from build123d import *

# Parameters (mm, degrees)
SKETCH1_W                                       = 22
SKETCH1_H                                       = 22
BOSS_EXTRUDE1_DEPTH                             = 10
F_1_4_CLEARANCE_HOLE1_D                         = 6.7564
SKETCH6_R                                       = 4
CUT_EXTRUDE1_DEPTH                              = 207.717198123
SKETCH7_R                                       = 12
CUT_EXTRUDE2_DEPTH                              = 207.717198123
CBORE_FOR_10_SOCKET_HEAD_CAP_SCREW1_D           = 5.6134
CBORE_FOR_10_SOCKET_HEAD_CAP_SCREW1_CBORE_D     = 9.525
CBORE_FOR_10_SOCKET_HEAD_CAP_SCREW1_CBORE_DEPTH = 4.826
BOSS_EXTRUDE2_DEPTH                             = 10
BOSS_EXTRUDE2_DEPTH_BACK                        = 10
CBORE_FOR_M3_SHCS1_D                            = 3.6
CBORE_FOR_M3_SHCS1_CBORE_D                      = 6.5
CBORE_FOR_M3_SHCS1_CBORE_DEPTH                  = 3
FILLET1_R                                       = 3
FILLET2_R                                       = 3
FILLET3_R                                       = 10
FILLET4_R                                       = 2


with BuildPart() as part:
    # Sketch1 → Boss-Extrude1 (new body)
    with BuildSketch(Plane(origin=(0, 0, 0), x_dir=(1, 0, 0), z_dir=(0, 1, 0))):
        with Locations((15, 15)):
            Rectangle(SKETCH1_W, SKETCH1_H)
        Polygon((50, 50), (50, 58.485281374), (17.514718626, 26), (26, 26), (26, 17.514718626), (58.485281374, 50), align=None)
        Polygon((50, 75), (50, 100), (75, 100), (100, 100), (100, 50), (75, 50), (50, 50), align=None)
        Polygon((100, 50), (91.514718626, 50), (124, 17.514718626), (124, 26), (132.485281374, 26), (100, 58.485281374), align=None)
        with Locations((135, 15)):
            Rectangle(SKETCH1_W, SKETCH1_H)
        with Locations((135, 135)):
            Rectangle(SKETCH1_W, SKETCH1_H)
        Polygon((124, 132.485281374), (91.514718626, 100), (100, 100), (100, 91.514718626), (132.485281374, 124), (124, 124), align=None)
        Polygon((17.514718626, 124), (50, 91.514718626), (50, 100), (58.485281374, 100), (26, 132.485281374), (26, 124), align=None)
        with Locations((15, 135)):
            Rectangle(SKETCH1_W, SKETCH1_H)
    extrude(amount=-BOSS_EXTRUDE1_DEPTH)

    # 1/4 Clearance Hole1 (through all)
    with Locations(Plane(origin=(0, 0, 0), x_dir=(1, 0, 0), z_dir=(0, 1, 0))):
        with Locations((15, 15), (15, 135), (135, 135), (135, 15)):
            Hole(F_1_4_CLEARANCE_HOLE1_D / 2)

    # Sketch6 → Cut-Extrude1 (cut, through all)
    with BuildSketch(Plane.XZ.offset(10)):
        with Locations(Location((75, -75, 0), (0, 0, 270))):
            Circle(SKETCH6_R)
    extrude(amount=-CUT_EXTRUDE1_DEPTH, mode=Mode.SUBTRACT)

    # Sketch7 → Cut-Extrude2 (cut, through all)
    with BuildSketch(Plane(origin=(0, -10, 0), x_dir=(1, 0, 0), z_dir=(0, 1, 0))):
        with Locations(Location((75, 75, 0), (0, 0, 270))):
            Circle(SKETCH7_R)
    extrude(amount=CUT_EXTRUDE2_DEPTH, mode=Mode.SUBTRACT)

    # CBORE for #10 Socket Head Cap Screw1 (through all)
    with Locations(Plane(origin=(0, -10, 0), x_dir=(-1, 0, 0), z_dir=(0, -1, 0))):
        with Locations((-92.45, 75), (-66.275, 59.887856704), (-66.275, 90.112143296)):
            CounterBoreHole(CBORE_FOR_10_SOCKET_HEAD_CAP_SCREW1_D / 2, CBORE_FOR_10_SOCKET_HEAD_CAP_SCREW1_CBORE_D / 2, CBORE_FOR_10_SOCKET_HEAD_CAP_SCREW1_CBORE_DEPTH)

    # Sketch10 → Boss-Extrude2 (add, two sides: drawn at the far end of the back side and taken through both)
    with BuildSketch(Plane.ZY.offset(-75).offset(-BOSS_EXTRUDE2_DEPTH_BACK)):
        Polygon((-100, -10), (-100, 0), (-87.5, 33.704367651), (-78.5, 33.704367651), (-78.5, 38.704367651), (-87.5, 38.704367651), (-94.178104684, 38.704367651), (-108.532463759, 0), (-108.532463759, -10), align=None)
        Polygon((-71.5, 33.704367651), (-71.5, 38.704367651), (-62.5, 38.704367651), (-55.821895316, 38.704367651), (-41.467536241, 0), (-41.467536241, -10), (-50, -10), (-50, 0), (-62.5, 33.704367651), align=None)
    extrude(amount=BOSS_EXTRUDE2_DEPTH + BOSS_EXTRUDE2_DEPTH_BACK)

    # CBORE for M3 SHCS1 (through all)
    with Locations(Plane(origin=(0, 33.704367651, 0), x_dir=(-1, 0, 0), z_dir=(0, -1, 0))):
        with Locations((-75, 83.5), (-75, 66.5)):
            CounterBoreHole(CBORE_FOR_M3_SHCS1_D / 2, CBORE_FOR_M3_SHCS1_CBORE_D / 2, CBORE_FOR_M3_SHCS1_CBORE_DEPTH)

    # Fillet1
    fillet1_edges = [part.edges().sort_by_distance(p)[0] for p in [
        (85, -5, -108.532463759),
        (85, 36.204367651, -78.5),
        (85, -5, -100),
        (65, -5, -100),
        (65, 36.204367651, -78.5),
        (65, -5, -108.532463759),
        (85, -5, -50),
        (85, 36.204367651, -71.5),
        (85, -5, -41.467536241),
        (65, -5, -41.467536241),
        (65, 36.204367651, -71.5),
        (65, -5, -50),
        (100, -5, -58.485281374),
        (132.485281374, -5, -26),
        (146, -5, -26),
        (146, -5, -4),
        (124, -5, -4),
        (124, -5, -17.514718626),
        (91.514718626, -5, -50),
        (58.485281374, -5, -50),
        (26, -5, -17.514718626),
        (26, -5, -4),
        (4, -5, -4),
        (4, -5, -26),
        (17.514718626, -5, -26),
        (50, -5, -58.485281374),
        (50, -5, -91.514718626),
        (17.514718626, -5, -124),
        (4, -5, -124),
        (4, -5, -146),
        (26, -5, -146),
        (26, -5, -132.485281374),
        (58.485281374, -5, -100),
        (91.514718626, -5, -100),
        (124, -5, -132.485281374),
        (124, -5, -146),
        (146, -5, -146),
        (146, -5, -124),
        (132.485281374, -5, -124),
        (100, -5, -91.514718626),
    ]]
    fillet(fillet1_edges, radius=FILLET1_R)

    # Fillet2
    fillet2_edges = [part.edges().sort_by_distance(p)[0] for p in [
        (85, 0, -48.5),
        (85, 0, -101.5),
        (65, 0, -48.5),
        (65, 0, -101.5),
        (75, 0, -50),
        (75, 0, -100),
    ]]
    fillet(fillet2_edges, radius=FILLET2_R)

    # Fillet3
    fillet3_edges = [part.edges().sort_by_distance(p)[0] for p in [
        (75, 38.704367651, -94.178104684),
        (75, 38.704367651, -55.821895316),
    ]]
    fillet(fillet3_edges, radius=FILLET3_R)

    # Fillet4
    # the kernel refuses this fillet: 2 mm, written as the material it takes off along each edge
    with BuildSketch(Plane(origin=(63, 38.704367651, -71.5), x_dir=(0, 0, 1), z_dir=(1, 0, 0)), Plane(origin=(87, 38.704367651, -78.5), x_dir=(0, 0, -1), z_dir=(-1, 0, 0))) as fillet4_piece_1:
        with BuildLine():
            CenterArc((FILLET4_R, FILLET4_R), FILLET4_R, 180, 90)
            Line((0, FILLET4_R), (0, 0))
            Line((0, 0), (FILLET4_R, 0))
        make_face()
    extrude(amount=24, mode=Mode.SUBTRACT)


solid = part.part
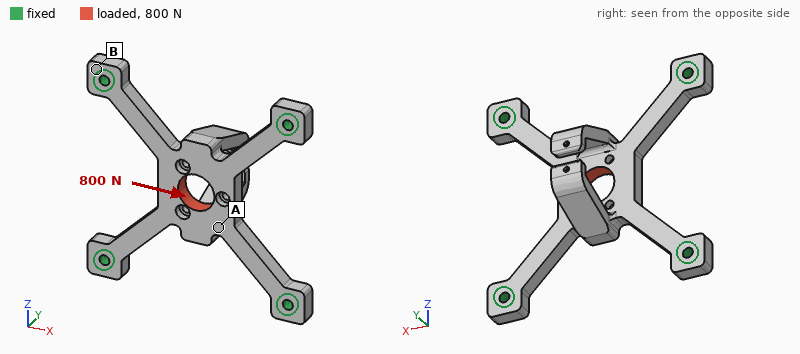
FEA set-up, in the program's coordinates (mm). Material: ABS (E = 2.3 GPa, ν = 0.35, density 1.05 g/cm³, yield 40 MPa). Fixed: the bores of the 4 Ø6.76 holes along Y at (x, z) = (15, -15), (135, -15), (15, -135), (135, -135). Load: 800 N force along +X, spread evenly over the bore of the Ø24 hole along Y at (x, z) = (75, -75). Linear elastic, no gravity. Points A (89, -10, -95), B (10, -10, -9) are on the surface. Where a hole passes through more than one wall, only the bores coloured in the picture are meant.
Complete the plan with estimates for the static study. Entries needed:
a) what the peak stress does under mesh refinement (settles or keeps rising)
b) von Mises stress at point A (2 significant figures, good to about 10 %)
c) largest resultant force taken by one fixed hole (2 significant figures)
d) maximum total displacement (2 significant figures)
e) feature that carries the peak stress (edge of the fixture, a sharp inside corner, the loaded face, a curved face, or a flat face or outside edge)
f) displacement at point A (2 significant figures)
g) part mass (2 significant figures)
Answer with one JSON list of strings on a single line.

["keeps rising", "1.5 MPa", "280 N", "0.12 mm", "a sharp inside corner", "0.085 mm", "77 g"]
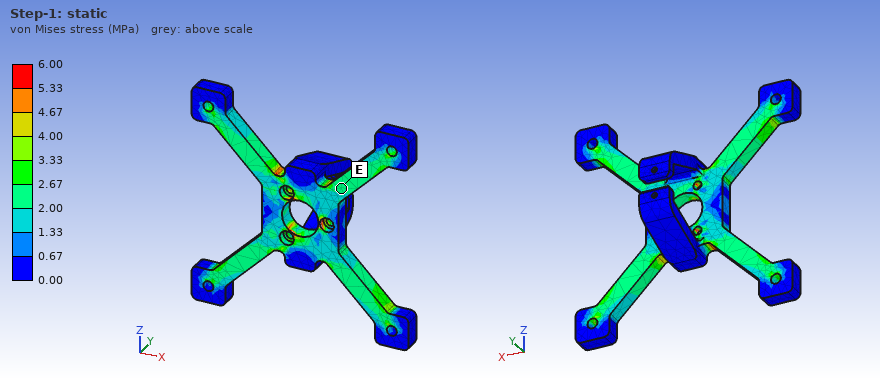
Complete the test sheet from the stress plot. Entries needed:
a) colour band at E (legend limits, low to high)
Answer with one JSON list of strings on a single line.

["2.00 to 2.67 MPa"]
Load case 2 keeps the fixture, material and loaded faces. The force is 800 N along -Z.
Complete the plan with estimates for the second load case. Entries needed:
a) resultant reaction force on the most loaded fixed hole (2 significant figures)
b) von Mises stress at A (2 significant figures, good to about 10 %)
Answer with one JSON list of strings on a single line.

["280 N", "1.9 MPa"]
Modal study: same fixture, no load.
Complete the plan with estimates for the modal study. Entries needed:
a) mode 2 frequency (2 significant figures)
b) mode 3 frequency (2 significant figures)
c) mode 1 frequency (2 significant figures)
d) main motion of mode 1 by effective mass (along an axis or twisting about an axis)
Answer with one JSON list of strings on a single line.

["600 Hz", "660 Hz", "440 Hz", "along Y"]
